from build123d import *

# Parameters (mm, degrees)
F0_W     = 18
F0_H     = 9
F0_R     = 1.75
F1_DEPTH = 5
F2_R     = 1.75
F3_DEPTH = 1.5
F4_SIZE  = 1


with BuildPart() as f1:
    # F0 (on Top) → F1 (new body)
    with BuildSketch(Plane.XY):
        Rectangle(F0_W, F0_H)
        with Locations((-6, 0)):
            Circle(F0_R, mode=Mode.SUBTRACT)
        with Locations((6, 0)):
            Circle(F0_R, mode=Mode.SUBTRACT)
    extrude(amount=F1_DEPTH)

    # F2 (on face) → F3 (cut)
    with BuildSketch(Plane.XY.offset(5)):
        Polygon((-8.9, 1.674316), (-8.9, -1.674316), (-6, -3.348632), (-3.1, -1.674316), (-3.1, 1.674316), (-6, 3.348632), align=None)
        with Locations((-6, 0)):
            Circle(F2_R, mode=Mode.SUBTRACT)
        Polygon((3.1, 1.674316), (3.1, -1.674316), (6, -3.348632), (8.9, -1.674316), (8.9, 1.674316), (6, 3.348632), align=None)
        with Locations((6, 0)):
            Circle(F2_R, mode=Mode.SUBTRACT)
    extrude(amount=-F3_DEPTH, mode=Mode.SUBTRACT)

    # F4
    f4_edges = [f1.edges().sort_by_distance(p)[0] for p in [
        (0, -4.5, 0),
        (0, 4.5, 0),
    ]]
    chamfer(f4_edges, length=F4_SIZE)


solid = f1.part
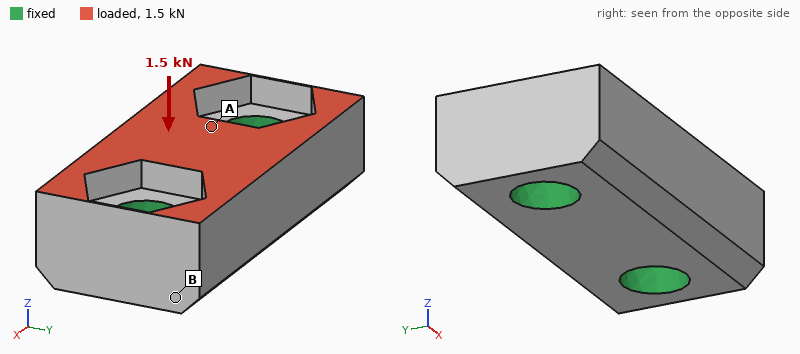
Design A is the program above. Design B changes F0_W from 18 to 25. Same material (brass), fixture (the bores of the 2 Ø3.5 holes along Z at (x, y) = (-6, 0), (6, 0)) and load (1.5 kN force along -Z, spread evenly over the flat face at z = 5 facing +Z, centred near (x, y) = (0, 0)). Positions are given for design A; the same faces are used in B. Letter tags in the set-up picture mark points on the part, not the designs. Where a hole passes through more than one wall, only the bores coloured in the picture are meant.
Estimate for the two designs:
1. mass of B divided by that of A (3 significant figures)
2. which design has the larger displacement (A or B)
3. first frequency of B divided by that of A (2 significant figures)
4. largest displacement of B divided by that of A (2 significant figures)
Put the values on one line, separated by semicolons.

1.48; B; 0.77; 1.4
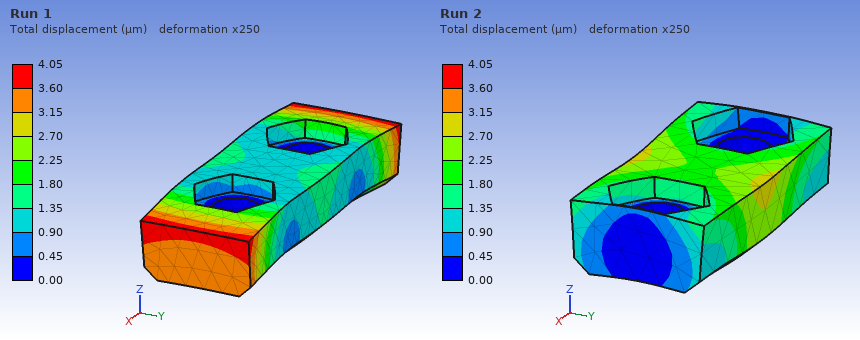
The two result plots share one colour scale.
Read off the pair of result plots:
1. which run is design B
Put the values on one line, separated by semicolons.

Run 1
